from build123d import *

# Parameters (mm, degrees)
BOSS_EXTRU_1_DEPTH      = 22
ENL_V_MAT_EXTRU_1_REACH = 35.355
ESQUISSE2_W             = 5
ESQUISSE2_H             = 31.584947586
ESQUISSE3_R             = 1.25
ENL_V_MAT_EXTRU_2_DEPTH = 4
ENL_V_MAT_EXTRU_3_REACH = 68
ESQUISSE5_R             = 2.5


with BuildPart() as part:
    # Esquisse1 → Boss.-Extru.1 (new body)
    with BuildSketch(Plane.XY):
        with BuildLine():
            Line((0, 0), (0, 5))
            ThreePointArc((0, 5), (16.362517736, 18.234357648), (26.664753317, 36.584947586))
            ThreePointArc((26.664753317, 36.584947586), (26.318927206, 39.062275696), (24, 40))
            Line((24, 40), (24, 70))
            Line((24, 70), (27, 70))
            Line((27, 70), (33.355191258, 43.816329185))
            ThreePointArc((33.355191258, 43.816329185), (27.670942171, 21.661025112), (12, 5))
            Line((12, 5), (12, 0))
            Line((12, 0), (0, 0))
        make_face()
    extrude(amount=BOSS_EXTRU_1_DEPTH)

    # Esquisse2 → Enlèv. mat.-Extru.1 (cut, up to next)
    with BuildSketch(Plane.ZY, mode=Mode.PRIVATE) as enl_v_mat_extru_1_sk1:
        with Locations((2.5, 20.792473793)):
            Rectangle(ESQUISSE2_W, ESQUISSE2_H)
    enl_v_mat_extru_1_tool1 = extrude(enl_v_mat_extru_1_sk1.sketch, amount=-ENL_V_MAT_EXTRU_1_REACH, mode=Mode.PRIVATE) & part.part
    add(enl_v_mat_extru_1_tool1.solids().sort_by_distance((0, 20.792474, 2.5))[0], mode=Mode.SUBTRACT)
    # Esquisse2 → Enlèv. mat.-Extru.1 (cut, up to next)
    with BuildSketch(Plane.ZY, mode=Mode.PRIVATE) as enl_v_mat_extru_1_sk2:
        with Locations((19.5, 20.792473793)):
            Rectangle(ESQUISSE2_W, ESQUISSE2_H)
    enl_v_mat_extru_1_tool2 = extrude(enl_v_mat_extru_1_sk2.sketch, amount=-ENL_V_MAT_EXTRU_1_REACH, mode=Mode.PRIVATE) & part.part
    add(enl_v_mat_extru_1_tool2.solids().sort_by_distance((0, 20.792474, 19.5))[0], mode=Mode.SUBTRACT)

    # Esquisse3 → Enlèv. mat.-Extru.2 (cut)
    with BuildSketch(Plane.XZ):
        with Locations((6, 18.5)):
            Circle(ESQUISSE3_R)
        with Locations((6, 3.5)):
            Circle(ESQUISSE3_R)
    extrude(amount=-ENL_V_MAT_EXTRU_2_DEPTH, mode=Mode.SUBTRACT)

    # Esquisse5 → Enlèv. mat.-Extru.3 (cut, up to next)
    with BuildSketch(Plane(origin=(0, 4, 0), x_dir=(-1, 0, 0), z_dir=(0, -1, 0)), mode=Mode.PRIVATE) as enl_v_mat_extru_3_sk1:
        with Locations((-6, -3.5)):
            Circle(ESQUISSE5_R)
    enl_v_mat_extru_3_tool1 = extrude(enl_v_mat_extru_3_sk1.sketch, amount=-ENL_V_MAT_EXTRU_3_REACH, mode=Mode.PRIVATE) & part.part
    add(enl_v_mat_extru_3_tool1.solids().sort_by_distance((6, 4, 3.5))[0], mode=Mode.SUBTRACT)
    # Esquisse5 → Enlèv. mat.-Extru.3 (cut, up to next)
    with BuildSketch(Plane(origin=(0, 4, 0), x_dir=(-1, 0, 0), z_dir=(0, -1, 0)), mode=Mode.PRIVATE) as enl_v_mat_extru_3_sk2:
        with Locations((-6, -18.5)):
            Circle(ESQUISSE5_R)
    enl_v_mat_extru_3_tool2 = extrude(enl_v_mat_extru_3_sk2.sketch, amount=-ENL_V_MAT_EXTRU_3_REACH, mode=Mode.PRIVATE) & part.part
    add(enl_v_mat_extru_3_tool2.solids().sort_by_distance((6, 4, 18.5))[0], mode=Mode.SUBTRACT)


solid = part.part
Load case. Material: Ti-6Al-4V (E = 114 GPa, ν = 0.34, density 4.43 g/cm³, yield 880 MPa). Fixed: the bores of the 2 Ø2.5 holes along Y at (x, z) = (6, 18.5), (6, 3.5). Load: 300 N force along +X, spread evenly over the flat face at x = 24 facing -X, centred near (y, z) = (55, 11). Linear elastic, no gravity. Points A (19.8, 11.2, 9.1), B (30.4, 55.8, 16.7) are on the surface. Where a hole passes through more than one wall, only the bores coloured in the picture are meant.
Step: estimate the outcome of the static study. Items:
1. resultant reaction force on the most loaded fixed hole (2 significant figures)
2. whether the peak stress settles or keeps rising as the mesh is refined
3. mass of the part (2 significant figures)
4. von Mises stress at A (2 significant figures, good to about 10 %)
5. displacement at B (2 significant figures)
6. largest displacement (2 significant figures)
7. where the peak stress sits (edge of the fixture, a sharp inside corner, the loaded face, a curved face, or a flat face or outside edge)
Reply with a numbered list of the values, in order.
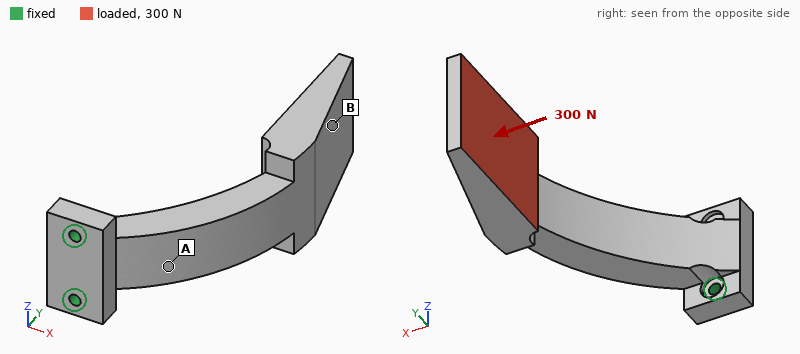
1. 230 N
2. keeps rising
3. 42 g
4. 110 MPa
5. 0.61 mm
6. 0.80 mm
7. edge of the fixture
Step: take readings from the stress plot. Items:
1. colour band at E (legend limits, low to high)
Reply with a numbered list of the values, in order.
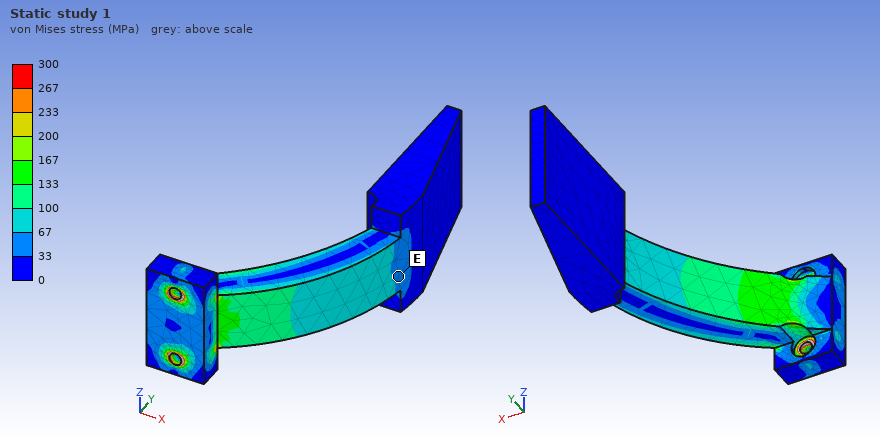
1. 33 to 67 MPa
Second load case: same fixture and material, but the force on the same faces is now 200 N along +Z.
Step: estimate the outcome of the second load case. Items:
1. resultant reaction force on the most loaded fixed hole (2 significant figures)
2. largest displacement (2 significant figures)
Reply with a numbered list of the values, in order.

1. 800 N
2. 0.24 mm
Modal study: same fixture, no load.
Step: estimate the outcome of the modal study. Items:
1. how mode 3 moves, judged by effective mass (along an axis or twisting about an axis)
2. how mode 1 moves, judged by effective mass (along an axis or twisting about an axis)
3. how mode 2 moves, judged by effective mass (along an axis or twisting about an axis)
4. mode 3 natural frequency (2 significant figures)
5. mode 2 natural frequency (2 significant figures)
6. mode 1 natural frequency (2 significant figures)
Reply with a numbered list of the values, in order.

1. along Y
2. along X
3. along Z
4. 3900 Hz
5. 1300 Hz
6. 790 Hz
